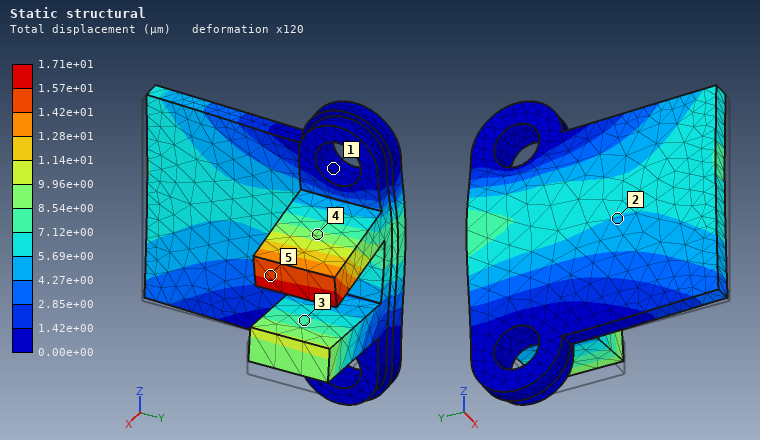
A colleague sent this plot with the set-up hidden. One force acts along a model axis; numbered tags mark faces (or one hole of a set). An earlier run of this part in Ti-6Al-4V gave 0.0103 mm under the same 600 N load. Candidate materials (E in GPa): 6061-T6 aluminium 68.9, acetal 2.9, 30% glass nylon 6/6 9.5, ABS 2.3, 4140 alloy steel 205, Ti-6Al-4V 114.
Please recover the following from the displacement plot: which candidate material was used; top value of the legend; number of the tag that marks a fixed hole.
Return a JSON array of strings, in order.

["6061-T6 aluminium", "1.71e+01 µm", "1"]
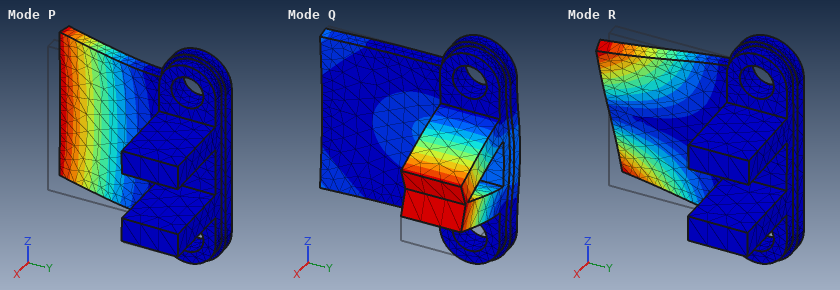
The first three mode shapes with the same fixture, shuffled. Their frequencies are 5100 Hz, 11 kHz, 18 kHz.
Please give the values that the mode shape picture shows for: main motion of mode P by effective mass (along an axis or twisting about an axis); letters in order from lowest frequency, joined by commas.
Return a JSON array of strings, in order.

["along X", "P, R, Q"]
